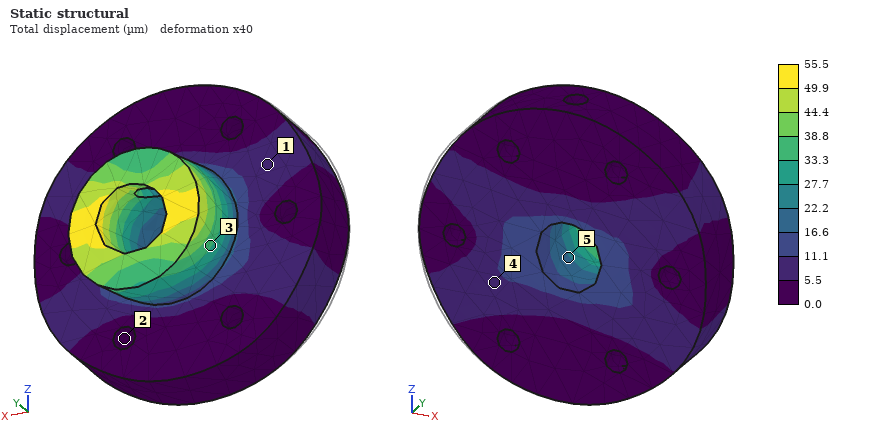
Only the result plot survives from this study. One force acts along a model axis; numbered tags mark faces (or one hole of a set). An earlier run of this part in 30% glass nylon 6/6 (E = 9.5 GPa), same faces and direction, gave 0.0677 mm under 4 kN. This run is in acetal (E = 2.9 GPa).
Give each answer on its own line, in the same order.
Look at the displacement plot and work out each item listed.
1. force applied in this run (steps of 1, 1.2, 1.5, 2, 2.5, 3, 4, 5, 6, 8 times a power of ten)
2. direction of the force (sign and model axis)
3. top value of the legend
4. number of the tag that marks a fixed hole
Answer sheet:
1 kN
+X
55.5 µm
2
